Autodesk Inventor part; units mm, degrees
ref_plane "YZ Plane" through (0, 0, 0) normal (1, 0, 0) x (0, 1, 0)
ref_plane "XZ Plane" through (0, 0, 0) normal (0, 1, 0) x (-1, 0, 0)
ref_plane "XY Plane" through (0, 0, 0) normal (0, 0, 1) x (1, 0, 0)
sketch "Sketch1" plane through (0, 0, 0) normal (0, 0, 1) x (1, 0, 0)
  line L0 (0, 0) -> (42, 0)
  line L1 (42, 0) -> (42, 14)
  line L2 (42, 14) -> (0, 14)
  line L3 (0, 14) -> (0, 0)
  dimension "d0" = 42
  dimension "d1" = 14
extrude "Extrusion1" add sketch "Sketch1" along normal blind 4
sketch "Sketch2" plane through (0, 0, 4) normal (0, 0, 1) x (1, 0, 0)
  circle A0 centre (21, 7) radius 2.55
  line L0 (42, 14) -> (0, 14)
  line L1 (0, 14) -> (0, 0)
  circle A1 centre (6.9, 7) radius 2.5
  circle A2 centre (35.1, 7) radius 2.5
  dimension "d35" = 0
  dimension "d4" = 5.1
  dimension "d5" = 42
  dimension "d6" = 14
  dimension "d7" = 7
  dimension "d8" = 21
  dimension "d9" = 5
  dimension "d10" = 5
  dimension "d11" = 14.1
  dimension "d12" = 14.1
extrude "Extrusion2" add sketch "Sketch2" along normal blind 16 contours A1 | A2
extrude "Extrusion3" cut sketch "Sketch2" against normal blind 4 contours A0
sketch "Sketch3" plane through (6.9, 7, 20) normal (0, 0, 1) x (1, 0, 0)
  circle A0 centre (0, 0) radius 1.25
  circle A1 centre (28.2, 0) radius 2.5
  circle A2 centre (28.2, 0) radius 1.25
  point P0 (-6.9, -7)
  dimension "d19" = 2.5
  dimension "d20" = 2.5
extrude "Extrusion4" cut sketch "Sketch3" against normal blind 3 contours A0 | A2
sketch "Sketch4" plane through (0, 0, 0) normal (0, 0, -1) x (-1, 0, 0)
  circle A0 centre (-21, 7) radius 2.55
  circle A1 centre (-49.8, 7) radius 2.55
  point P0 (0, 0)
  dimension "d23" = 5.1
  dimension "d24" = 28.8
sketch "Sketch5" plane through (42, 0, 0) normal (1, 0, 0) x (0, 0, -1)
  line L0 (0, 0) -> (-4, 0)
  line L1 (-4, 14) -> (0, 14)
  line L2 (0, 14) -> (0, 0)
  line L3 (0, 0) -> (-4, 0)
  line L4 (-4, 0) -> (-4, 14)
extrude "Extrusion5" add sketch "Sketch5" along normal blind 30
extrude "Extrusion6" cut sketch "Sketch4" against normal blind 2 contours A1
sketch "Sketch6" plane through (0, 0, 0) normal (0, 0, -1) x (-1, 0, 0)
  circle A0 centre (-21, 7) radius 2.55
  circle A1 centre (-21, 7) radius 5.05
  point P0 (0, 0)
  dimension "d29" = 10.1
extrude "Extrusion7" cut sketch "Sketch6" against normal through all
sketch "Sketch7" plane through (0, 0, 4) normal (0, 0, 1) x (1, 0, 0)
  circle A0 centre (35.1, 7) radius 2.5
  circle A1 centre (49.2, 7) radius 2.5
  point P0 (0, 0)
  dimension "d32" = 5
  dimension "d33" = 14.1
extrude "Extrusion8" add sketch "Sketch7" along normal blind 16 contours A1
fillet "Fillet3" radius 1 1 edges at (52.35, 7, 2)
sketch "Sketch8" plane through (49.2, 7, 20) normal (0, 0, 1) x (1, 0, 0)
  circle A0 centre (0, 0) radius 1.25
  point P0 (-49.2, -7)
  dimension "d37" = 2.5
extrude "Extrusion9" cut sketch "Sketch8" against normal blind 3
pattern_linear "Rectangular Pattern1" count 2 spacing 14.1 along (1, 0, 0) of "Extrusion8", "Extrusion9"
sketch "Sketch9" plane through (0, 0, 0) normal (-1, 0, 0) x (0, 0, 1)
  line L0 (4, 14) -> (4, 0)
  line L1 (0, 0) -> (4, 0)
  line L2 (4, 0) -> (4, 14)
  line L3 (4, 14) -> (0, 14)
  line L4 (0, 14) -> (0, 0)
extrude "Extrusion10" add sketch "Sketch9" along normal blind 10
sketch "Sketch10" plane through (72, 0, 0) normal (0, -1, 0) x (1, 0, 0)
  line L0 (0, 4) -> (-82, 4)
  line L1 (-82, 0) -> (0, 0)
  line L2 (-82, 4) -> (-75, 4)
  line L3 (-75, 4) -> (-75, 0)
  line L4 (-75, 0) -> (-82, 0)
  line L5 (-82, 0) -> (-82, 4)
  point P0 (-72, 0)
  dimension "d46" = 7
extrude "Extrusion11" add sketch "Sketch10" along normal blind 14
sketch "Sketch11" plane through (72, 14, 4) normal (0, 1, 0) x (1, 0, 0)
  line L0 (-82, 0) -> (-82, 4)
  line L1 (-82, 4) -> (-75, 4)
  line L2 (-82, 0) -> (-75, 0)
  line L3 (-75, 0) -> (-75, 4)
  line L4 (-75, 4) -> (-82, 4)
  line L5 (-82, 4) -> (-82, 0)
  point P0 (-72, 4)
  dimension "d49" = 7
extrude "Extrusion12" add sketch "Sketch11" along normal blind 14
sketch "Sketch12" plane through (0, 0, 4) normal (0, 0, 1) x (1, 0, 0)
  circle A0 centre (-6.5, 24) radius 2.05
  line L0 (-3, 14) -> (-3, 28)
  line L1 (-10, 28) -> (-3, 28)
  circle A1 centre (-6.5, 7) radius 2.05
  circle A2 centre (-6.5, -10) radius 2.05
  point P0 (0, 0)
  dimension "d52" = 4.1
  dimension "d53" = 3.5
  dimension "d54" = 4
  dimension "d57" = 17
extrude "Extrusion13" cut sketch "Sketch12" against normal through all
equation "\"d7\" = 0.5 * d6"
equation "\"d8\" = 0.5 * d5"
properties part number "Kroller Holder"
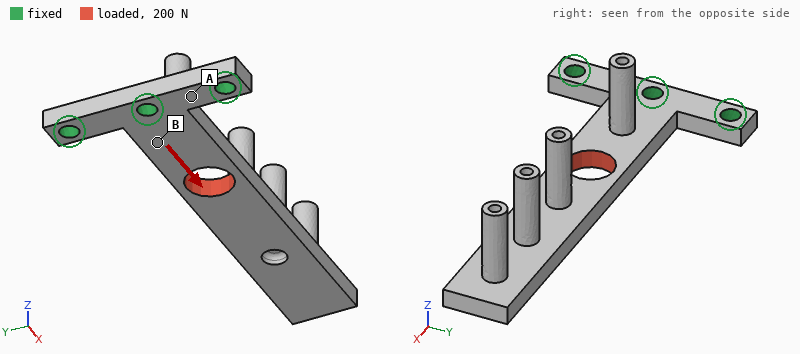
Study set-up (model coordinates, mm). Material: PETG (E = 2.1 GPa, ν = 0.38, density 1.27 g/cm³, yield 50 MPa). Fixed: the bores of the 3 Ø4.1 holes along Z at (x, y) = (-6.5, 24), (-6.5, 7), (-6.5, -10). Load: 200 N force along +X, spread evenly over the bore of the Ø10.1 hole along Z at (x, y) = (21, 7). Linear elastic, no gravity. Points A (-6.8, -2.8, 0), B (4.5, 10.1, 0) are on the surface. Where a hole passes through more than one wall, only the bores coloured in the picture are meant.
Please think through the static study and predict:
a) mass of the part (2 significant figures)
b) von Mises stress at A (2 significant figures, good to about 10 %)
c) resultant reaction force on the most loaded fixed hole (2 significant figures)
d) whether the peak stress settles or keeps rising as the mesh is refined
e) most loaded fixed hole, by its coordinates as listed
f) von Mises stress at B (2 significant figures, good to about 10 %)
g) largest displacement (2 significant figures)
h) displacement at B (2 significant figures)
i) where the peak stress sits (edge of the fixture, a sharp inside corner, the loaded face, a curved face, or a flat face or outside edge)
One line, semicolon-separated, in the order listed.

7.7 g; 1.2 MPa; 180 N; keeps rising; (-6.5, 7); 3.7 MPa; 84 µm; 20 µm; a sharp inside corner
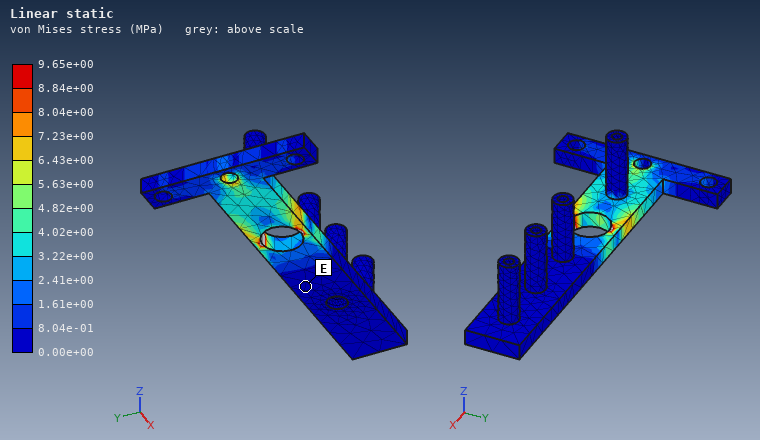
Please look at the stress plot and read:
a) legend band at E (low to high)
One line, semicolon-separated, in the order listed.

0.00e+00 to 8.04e-01 MPa
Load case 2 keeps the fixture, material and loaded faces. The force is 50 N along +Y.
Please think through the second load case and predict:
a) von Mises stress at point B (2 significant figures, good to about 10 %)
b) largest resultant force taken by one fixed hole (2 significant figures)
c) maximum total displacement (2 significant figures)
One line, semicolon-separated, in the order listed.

3.5 MPa; 39 N; 0.97 mm
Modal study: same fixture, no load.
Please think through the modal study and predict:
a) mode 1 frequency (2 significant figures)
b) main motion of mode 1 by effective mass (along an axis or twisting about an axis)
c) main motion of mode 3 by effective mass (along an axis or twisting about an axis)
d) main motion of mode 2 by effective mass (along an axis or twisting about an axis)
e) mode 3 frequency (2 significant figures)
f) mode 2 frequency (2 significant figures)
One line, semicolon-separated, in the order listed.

100 Hz; along Z; twisting about X; along Y; 680 Hz; 350 Hz
